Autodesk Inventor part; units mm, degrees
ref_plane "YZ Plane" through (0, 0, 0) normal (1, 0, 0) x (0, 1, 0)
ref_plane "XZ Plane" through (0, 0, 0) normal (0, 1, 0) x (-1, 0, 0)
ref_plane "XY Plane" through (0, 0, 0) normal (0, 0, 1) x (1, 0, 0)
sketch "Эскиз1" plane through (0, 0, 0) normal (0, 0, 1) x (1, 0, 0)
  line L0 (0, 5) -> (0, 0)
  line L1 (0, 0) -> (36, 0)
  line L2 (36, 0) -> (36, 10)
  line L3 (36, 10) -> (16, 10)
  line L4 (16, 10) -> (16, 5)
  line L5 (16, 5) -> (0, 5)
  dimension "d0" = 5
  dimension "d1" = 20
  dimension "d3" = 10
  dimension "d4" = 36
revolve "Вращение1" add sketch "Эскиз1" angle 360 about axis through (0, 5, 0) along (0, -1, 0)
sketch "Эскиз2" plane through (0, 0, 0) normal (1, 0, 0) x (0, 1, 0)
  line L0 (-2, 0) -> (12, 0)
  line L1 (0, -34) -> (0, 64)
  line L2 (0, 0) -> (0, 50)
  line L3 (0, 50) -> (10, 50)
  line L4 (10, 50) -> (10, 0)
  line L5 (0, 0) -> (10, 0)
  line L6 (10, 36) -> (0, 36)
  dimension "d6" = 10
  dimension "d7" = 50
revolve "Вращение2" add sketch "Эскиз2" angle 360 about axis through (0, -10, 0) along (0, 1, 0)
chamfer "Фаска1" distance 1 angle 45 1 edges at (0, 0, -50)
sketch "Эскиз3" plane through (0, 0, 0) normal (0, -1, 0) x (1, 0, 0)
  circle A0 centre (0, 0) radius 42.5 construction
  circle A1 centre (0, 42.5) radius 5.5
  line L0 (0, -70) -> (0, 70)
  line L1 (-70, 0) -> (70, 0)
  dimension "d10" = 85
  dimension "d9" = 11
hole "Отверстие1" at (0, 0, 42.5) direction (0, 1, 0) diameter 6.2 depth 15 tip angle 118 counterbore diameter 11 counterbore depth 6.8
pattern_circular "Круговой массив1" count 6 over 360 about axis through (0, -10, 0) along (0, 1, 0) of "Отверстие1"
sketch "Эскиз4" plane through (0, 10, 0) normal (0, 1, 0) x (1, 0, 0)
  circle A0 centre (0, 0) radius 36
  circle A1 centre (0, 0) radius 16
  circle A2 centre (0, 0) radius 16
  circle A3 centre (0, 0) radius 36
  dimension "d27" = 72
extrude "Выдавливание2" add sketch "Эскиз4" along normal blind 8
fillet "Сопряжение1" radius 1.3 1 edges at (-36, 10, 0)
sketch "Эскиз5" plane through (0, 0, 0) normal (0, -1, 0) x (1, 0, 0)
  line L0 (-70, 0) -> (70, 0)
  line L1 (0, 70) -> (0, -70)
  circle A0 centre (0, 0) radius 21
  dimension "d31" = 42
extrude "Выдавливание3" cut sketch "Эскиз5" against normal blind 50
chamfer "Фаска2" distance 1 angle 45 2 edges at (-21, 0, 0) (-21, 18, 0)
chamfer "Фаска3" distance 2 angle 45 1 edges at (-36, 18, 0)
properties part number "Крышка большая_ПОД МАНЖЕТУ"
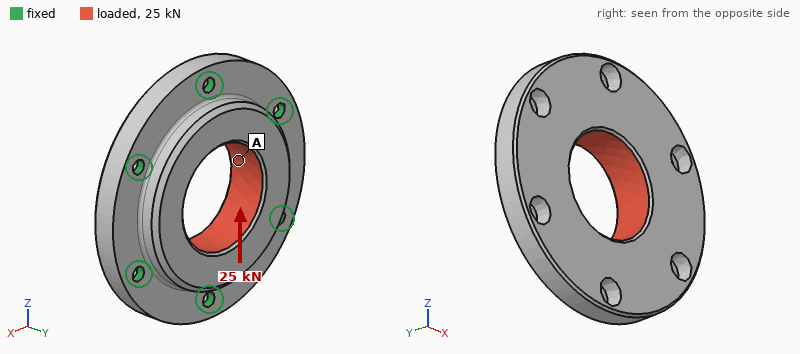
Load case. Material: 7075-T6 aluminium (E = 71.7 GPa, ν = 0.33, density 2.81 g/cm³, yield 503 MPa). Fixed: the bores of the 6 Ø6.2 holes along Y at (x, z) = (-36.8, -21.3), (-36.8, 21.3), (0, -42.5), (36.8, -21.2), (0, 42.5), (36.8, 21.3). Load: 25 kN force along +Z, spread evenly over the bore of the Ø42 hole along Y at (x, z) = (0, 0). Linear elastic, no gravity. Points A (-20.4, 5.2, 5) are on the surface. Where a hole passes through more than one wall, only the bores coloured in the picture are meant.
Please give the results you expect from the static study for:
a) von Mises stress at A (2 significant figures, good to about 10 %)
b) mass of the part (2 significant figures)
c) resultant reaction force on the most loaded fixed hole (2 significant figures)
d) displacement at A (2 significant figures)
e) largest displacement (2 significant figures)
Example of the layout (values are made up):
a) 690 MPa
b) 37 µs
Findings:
a) 21 MPa
b) 230 g
c) 5.1 kN
d) 11 µm
e) 13 µm
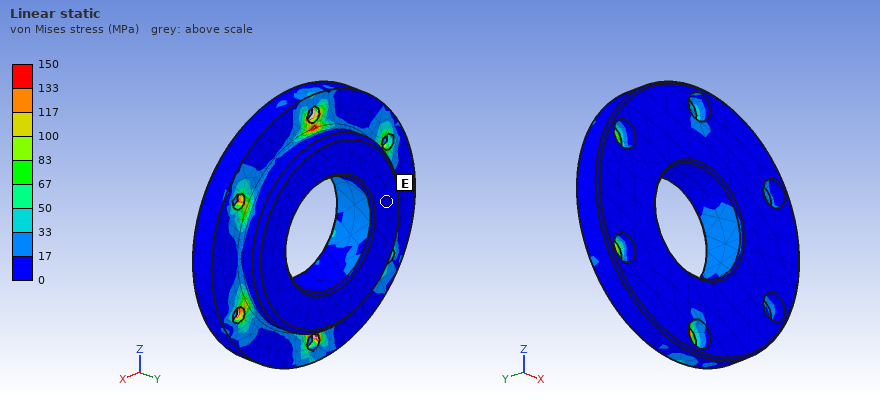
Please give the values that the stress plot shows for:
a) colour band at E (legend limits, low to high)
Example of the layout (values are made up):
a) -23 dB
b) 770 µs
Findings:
a) 0 to 17 MPa
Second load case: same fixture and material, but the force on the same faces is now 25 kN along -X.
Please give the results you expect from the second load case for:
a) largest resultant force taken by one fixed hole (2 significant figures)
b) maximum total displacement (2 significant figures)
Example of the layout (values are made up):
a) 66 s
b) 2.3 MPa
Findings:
a) 4.7 kN
b) 13 µm
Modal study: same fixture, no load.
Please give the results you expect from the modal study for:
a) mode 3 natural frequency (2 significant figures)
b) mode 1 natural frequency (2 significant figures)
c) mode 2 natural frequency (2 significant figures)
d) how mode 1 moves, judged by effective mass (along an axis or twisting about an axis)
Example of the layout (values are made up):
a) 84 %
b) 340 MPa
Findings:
a) 14 kHz
b) 10 kHz
c) 14 kHz
d) along Y
